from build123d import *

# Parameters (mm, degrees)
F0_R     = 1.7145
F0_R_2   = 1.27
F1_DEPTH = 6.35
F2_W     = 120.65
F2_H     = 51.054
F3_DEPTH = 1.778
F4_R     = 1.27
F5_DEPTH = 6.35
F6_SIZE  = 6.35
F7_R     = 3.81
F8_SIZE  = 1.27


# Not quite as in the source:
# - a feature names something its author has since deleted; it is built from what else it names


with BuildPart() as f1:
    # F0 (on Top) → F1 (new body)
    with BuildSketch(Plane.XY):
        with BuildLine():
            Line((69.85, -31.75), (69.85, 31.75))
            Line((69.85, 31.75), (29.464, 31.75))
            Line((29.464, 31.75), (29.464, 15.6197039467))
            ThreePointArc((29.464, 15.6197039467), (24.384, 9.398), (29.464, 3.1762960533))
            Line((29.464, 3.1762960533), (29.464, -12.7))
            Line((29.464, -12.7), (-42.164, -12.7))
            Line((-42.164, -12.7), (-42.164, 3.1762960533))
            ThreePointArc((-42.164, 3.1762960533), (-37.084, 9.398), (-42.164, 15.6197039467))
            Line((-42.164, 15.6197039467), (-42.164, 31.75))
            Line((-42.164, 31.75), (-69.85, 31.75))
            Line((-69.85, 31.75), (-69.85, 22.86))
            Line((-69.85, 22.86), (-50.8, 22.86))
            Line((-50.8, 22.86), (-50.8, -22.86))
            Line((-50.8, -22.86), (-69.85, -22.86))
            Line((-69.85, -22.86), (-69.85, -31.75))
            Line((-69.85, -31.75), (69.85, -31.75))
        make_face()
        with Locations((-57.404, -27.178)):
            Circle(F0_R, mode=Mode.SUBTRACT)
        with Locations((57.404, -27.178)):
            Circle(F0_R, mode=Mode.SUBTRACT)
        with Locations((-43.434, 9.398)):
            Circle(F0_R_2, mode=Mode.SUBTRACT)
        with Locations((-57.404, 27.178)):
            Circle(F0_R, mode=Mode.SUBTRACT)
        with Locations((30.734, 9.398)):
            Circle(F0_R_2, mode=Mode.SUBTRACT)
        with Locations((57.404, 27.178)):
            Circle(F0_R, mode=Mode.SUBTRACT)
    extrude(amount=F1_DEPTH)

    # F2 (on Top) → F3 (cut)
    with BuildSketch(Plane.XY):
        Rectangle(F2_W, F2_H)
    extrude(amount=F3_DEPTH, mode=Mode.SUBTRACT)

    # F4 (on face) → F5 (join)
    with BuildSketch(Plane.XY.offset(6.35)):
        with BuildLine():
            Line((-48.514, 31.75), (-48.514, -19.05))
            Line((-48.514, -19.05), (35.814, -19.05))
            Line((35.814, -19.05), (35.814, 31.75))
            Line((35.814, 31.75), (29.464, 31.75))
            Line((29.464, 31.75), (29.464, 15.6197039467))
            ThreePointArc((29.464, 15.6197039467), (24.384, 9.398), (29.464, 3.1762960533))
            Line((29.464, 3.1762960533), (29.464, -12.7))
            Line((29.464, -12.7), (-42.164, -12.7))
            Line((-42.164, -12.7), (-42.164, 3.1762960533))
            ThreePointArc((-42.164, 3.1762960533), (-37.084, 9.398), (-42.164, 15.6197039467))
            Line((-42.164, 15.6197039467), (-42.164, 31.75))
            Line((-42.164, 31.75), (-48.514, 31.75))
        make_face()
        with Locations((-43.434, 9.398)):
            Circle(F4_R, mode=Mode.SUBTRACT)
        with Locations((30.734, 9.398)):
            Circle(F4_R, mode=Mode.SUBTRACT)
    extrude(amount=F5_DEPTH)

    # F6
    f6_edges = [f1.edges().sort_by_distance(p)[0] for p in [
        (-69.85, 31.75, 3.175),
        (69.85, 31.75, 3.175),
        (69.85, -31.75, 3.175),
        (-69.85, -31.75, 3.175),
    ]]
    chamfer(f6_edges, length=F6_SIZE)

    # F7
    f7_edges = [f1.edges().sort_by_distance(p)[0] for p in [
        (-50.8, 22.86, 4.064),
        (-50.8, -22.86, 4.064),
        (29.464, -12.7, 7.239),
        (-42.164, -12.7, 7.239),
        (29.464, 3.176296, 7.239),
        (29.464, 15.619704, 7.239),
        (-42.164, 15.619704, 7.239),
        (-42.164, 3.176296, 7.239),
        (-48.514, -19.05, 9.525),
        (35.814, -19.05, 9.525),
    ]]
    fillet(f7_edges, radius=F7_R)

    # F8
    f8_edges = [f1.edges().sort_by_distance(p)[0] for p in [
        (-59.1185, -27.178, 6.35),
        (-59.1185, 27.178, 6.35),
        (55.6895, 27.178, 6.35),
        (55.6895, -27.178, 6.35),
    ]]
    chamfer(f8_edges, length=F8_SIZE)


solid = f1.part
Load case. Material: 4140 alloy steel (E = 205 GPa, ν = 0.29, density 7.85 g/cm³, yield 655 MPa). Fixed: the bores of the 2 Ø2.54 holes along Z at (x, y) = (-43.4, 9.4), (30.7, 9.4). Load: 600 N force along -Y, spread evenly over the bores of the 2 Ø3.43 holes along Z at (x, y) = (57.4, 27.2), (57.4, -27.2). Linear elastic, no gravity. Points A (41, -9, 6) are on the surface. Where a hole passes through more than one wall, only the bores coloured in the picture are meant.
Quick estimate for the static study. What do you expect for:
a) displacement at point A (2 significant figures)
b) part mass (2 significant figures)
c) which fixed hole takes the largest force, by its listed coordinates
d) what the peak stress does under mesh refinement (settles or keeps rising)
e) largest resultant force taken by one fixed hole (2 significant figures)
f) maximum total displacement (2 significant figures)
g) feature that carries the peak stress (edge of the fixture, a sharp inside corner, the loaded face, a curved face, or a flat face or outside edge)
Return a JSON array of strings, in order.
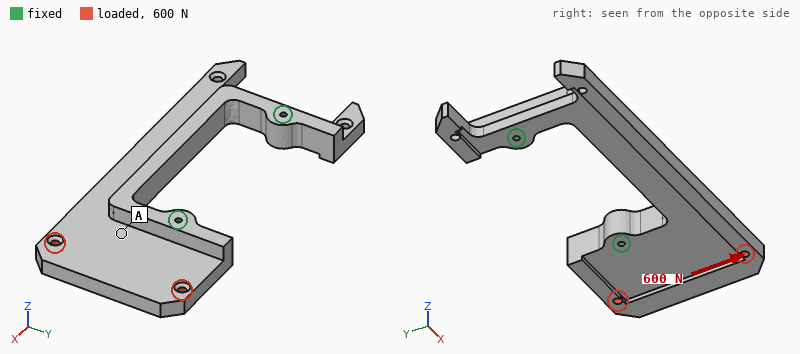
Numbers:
["5.6 µm", "260 g", "(30.7, 9.4)", "keeps rising", "750 N", "16 µm", "edge of the fixture"]
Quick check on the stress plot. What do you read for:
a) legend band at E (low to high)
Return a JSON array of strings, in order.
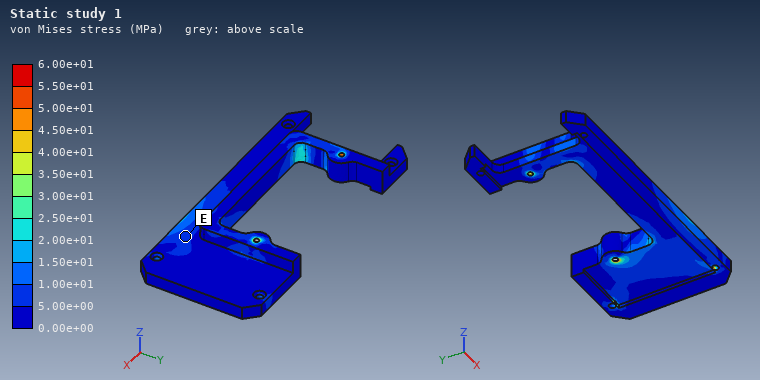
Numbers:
["5.00e+00 to 1.00e+01 MPa"]
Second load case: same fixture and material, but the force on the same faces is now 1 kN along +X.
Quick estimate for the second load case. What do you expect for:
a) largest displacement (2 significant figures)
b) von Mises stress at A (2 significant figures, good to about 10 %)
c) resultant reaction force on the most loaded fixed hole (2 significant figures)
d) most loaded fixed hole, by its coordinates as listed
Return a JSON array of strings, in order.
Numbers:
["11 µm", "7.1 MPa", "870 N", "(30.7, 9.4)"]
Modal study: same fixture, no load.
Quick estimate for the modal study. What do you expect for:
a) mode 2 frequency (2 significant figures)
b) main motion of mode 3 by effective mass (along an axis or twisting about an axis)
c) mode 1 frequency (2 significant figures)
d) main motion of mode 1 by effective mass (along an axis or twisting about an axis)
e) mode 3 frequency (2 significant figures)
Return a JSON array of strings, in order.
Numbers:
["2300 Hz", "along X", "2200 Hz", "along Z", "3100 Hz"]
